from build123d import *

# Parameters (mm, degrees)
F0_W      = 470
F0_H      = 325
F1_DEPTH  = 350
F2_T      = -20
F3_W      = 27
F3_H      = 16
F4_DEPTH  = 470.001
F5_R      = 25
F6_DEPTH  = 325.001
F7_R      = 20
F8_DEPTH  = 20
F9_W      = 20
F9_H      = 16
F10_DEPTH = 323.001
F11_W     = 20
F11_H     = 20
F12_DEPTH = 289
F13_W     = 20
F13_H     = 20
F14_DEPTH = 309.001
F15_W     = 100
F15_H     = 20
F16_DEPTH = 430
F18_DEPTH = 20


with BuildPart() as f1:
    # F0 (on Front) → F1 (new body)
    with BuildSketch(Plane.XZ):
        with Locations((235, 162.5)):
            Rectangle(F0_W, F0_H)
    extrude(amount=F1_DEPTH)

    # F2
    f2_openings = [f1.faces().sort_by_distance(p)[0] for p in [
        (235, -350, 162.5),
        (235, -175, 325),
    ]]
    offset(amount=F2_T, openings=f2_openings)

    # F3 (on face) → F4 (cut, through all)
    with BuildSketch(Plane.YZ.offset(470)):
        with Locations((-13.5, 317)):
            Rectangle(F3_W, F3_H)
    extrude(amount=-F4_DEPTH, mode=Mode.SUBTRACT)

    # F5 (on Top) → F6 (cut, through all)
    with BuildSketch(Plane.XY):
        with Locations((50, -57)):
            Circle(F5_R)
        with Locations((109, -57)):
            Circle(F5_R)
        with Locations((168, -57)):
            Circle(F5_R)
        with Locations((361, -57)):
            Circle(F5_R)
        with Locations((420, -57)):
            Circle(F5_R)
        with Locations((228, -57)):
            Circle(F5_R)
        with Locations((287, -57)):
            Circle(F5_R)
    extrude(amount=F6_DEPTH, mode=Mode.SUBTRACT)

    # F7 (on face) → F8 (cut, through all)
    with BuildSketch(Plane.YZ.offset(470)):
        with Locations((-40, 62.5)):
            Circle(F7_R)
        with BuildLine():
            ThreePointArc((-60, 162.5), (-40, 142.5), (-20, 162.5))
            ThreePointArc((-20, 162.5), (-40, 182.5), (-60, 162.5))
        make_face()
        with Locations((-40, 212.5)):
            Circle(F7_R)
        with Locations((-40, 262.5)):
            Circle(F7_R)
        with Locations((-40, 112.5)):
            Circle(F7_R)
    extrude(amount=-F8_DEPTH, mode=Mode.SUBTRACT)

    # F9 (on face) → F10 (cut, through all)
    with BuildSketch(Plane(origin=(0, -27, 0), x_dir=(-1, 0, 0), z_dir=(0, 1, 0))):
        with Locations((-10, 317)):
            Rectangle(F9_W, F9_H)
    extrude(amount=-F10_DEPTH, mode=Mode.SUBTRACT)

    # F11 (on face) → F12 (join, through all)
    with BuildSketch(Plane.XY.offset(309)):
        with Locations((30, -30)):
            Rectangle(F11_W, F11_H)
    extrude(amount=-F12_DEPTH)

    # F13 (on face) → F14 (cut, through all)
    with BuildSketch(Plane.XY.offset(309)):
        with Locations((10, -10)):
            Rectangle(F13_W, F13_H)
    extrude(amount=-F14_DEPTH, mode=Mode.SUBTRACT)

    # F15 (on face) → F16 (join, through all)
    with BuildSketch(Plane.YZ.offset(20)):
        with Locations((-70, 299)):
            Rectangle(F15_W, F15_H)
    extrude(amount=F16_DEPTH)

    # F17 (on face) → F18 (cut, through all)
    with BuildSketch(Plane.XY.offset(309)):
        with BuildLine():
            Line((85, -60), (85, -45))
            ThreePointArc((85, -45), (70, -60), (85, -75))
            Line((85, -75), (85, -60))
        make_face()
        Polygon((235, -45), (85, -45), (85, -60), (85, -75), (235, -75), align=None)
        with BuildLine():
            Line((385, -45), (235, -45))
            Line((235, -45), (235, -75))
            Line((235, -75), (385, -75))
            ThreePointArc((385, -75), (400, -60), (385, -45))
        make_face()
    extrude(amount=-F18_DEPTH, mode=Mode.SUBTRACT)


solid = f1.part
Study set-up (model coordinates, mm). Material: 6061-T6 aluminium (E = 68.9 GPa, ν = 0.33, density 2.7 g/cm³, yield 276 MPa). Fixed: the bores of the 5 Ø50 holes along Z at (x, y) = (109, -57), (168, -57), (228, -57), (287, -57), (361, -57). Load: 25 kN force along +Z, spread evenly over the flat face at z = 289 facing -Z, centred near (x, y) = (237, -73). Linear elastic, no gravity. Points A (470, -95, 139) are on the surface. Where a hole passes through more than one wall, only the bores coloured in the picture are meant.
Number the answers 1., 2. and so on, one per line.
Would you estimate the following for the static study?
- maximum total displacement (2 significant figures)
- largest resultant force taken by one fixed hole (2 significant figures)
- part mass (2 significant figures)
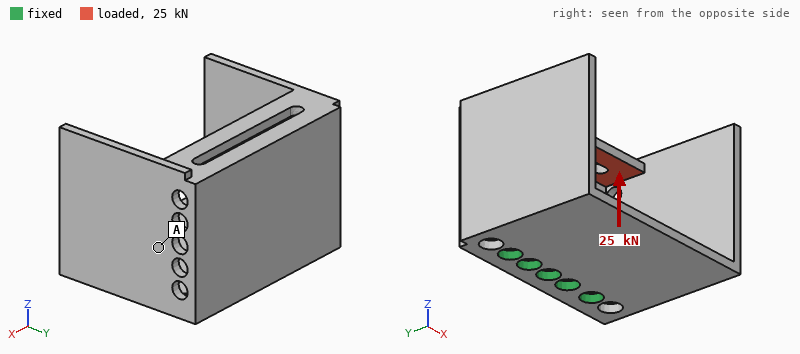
1. 1.6 mm
2. 11 kN
3. 27 kg
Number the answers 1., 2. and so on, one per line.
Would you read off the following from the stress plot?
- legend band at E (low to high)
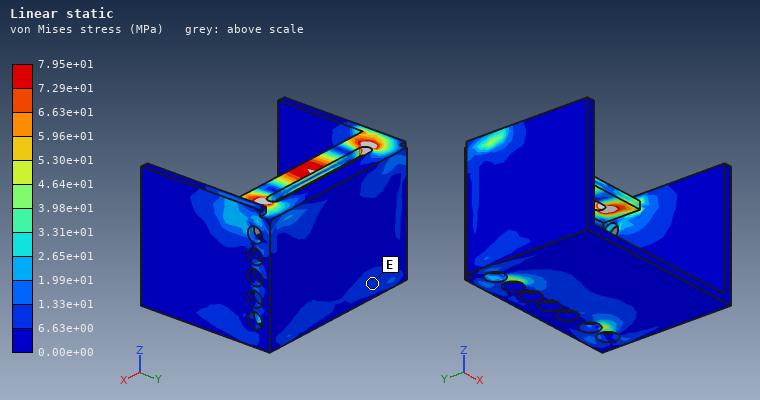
1. 6.63e+00 to 1.33e+01 MPa
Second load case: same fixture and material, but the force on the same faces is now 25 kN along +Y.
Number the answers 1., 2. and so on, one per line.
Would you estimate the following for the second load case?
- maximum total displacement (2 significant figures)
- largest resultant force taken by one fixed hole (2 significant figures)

1. 3.1 mm
2. 19 kN
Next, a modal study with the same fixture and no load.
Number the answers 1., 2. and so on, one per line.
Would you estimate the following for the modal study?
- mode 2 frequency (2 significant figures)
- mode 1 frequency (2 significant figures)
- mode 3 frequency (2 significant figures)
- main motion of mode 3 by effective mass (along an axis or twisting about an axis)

1. 210 Hz
2. 150 Hz
3. 330 Hz
4. along X
